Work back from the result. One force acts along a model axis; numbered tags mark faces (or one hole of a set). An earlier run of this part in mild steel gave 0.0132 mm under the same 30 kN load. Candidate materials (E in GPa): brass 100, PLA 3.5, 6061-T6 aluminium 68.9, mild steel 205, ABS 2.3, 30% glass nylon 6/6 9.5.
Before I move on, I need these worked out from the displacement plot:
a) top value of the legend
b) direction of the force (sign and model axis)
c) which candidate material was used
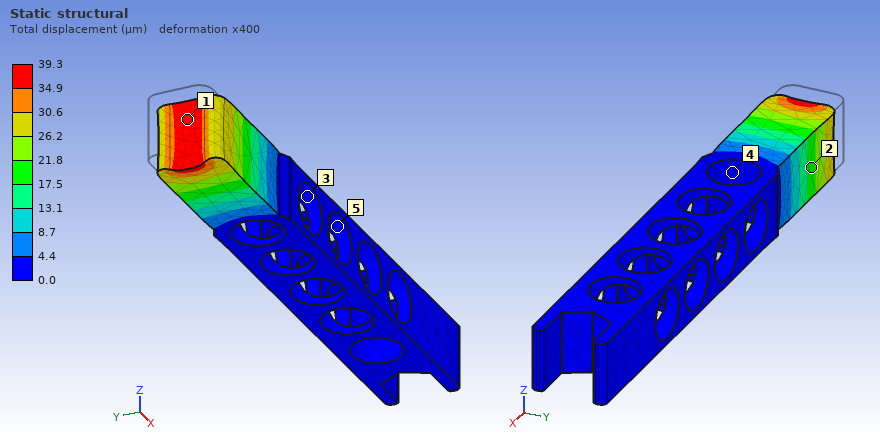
39.3 µm
+X
6061-T6 aluminium
